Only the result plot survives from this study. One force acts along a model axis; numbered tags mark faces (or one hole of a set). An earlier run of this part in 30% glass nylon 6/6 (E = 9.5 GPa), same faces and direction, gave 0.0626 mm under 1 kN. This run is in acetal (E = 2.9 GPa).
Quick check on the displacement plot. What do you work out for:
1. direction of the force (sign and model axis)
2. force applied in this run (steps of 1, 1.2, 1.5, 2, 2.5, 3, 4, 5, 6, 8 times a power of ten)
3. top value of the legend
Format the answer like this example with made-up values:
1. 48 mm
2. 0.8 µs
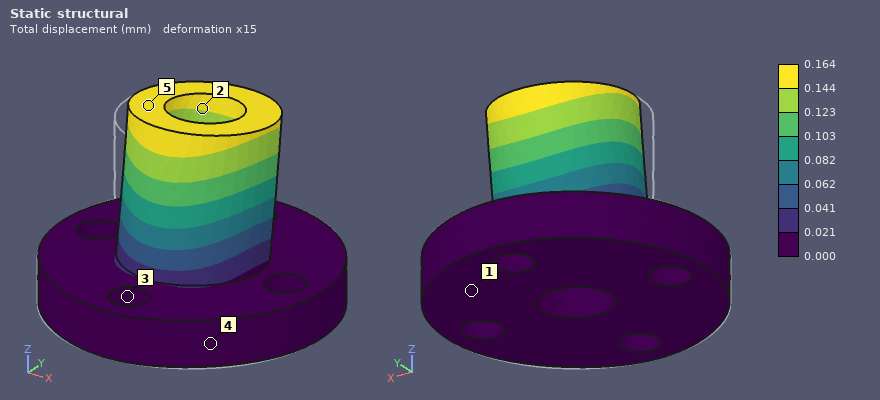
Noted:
1. +Y
2. 800 N
3. 0.164 mm
